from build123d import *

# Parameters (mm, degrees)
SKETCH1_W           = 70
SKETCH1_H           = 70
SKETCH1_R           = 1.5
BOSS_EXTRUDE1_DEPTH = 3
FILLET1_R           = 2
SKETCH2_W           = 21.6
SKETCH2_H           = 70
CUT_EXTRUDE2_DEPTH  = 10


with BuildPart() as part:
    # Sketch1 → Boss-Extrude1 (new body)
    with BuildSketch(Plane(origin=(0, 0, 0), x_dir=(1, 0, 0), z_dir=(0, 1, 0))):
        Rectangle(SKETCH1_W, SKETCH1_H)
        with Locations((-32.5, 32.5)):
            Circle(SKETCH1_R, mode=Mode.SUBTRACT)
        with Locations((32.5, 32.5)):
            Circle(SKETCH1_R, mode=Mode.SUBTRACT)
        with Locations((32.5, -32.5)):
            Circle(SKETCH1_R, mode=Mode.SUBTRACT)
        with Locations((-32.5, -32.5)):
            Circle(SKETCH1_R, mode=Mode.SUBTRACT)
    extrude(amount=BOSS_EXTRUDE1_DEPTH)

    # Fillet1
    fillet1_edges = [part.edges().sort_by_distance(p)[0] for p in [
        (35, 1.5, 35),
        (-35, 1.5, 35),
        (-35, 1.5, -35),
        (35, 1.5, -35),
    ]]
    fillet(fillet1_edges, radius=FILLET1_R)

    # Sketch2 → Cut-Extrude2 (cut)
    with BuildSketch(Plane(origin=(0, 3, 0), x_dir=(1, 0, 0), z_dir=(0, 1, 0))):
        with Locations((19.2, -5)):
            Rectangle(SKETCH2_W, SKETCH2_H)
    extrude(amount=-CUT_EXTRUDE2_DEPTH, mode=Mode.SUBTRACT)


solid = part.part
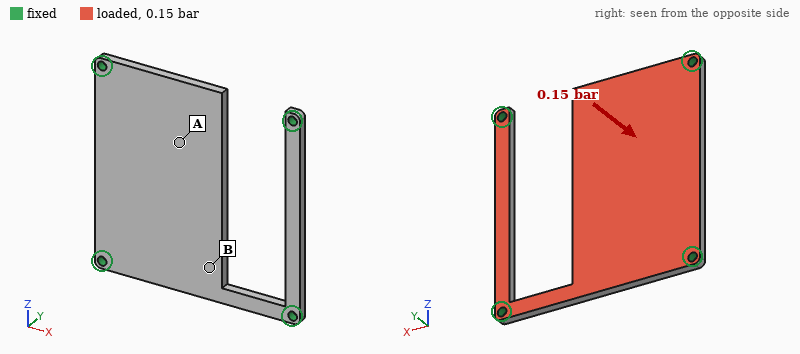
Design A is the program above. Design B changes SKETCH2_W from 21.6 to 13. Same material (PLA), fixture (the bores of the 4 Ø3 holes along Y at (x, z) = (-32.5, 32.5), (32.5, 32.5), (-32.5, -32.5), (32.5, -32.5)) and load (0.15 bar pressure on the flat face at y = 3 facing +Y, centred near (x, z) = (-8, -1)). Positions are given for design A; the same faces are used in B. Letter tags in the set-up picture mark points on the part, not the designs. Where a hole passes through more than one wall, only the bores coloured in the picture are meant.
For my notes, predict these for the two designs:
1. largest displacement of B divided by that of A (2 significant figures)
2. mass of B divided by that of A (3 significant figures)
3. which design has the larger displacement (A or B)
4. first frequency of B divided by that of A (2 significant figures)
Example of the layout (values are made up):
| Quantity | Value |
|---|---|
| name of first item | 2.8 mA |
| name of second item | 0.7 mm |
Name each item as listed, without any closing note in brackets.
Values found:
| Quantity | Value |
|---|---|
| largest displacement of B divided by that of A | 1.2 |
| mass of B divided by that of A | 1.16 |
| which design has the larger displacement | B |
| first frequency of B divided by that of A | 0.92 |
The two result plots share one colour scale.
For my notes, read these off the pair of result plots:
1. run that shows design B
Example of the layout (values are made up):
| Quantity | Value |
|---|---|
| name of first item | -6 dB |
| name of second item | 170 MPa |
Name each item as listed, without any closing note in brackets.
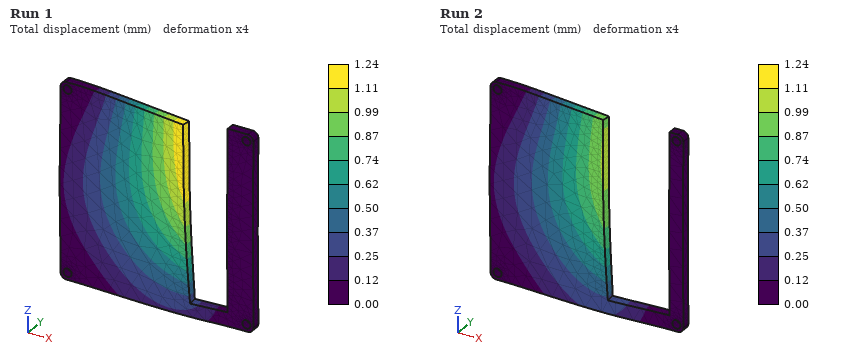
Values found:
| Quantity | Value |
|---|---|
| run that shows design B | Run 1 |
